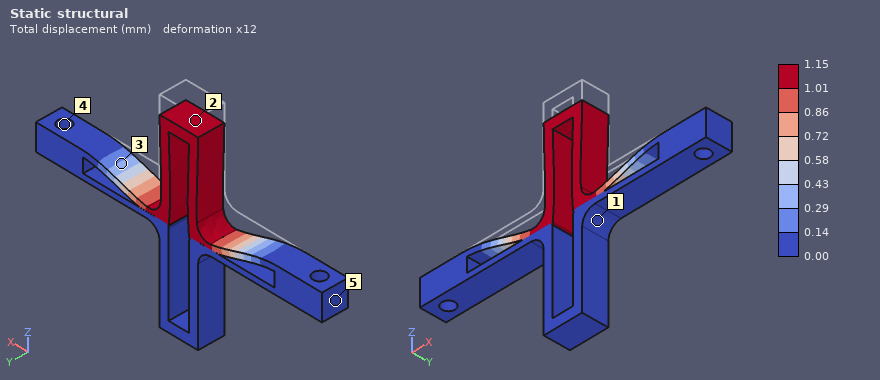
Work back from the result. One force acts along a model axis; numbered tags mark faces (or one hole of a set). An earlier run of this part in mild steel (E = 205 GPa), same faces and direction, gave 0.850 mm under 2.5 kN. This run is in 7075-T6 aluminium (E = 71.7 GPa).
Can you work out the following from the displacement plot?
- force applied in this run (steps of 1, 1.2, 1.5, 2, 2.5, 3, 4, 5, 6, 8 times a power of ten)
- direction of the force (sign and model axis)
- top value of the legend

1.2 kN
-Z
1.15 mm
